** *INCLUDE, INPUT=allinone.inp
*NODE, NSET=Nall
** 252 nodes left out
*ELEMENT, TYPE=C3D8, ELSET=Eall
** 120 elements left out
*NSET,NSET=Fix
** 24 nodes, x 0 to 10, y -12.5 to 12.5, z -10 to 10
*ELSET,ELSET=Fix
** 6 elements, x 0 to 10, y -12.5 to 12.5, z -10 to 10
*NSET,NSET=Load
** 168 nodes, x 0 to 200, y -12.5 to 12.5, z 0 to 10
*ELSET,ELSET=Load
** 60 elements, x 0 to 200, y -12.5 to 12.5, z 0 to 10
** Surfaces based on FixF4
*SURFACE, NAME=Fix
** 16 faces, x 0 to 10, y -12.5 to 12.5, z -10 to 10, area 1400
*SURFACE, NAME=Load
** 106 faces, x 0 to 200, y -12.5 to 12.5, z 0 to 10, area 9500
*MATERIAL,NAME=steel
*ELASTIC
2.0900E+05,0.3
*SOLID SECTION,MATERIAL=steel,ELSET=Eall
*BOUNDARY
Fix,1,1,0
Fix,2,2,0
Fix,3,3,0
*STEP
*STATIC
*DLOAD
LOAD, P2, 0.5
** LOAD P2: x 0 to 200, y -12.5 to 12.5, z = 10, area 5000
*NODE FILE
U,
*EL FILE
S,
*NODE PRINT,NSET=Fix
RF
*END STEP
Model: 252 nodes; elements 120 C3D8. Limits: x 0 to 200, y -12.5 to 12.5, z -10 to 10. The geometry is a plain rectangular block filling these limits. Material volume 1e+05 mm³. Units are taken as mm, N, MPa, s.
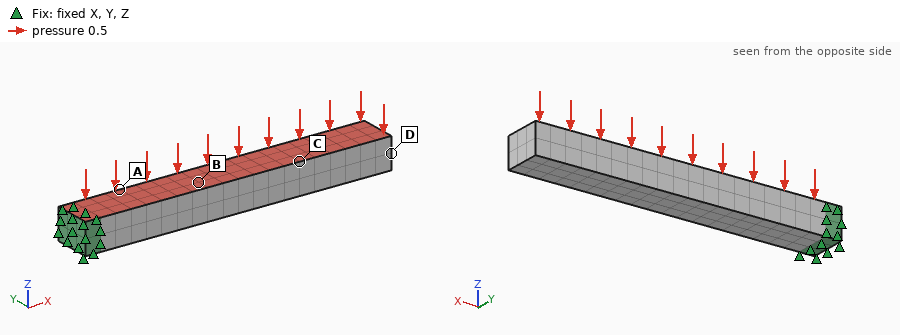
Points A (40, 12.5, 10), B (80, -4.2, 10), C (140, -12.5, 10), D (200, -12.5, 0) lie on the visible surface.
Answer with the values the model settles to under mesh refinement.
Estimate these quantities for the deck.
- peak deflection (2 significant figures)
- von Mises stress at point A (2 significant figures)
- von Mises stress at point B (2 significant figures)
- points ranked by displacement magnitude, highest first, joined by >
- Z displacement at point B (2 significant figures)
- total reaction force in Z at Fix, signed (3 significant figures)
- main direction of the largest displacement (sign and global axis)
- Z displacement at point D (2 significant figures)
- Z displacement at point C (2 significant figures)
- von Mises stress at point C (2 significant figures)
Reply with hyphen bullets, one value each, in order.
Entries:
- 0.59 mm
- 96 MPa
- 54 MPa
- D > C > B > A
- -0.13 mm
- 2500 N
- -Z
- -0.58 mm
- -0.34 mm
- 14 MPa
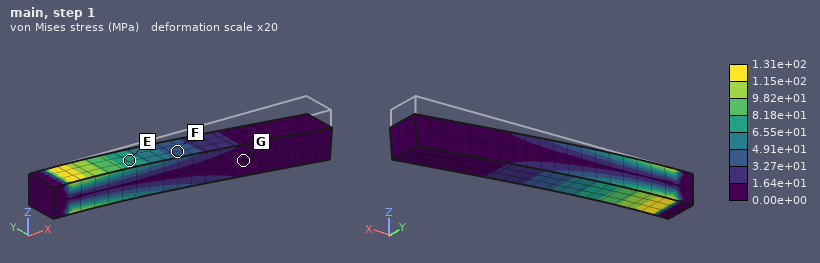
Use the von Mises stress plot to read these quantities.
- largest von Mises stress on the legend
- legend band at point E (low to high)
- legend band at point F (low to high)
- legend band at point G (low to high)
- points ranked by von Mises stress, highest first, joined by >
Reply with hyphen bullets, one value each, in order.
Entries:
- 1.31e+02 MPa
- 6.55e+01 to 8.18e+01 MPa
- 3.27e+01 to 4.91e+01 MPa
- 0.00e+00 to 1.64e+01 MPa
- E > F > G
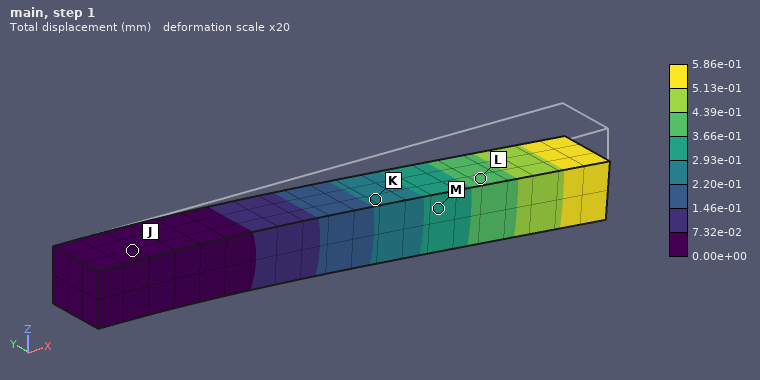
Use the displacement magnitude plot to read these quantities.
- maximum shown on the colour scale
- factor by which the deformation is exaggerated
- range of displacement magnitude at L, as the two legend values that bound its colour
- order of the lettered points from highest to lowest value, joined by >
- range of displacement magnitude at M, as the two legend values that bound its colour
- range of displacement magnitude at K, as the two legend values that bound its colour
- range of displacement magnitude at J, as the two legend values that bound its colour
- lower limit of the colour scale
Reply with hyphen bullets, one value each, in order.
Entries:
- 5.86e-01 mm
- 20
- 3.66e-01 to 4.39e-01 mm
- L > M > K > J
- 2.93e-01 to 3.66e-01 mm
- 2.20e-01 to 2.93e-01 mm
- 0.00e+00 to 7.32e-02 mm
- 0.00e+00 mm
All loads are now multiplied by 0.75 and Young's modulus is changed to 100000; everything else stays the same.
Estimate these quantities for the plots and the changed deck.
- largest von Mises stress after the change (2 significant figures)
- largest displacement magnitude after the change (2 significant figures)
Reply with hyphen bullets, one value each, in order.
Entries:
- 98 MPa
- 0.92 mm
